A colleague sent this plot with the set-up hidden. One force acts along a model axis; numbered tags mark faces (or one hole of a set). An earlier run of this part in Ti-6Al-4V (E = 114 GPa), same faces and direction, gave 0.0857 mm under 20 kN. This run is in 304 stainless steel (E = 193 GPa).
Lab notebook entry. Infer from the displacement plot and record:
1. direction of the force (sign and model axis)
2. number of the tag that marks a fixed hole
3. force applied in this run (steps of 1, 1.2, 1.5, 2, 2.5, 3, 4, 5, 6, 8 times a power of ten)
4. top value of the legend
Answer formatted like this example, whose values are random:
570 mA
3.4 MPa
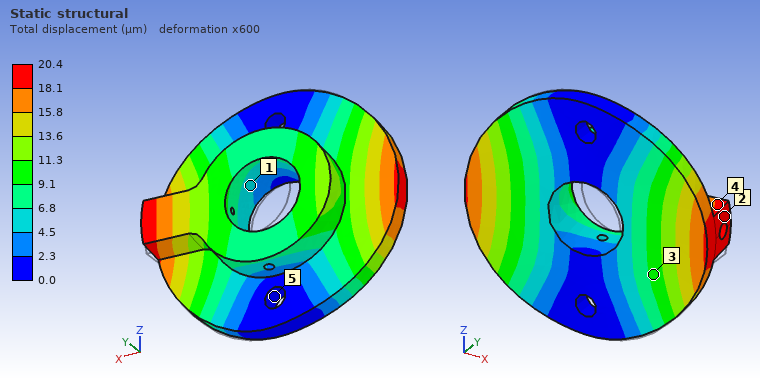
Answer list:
-X
5
8 kN
20.4 µm
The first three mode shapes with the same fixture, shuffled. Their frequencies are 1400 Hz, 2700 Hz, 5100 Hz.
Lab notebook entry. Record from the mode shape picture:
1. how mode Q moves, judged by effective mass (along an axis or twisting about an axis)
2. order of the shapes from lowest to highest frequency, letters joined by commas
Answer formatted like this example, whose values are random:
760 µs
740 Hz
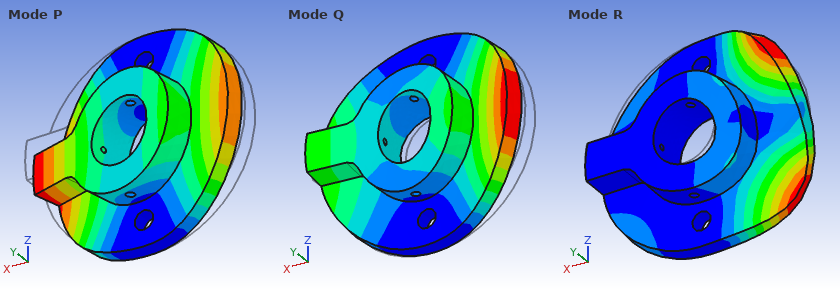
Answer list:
along Y
P, Q, R
